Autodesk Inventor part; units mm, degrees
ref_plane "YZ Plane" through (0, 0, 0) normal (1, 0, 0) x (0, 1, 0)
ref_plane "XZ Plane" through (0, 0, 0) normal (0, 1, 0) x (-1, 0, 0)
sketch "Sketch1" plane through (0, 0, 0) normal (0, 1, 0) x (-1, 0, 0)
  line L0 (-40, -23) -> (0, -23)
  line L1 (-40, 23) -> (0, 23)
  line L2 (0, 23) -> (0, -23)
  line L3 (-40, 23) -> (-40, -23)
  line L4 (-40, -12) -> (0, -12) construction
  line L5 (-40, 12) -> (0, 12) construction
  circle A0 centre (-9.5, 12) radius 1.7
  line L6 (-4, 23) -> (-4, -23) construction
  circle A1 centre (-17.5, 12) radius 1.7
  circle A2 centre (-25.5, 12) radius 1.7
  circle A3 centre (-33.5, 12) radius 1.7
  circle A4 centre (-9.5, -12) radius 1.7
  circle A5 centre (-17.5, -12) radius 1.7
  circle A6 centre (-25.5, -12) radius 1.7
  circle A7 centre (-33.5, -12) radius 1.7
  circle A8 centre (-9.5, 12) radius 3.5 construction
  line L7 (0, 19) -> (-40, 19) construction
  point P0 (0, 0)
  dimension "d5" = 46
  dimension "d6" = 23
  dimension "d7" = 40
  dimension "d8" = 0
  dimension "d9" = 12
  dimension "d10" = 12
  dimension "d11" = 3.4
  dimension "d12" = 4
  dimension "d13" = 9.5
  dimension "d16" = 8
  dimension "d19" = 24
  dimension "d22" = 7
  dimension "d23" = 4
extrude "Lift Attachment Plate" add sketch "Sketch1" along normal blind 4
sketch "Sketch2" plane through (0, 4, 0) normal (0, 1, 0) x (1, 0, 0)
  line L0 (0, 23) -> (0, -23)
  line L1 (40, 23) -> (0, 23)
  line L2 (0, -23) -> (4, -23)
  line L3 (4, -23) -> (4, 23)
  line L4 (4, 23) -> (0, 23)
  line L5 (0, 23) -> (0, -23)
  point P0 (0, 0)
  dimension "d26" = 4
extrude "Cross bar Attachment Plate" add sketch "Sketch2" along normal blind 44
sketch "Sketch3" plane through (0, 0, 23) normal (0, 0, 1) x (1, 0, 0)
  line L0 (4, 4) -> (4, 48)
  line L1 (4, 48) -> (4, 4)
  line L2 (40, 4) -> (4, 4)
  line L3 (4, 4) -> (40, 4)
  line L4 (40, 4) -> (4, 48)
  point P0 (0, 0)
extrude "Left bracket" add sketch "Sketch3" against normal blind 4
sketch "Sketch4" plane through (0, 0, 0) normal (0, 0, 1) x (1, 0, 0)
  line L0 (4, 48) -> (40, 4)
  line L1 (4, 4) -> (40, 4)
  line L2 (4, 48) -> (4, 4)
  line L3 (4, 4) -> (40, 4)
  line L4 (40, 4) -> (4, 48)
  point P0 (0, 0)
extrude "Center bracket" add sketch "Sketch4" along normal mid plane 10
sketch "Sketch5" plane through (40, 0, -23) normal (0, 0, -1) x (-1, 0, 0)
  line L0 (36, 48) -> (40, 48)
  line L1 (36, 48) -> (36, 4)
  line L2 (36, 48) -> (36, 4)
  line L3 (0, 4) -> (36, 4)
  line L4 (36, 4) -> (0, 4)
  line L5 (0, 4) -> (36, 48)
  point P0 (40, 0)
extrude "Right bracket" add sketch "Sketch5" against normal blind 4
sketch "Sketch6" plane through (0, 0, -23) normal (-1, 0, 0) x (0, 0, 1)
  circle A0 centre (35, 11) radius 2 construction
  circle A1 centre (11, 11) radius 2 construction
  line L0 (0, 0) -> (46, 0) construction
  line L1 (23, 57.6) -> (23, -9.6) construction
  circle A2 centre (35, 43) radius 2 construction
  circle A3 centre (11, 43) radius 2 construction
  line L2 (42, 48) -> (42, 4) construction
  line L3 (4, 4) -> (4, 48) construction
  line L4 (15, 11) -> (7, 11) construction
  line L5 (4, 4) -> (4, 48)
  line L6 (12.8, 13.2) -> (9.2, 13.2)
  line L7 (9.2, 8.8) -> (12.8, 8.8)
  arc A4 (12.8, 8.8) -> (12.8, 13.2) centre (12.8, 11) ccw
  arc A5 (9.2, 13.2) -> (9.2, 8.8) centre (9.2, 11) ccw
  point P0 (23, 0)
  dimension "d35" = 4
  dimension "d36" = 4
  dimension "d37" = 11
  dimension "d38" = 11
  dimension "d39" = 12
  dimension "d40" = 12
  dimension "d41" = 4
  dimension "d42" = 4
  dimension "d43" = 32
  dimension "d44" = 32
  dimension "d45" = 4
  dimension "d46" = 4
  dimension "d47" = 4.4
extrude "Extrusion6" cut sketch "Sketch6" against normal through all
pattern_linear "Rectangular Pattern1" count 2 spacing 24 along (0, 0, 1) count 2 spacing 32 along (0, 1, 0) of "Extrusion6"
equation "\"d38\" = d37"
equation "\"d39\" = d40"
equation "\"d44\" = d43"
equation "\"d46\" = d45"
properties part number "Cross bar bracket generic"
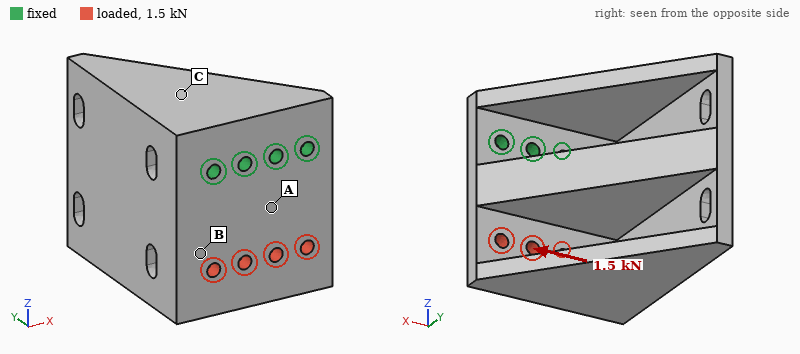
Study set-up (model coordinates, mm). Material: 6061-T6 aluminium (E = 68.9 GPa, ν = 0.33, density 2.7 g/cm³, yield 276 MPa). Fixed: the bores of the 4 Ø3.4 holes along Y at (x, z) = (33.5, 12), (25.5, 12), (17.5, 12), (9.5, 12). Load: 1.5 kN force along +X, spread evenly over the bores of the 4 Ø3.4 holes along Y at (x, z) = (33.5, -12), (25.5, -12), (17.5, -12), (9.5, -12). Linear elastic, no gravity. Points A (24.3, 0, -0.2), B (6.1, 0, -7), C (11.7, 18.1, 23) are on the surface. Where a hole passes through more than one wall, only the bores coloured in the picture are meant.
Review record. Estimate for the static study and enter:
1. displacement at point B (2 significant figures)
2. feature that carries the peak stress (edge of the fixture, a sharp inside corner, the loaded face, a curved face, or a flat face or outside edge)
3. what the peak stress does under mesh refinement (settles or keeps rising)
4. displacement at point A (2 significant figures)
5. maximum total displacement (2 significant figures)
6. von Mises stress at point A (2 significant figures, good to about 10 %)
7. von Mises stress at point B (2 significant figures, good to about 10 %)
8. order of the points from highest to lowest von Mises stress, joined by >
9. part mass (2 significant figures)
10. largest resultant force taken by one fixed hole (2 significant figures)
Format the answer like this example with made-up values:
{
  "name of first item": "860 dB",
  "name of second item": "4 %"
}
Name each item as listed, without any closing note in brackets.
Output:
{
  "displacement at point B": "13 µm",
  "feature that carries the peak stress": "edge of the fixture",
  "what the peak stress does under mesh refinement": "keeps rising",
  "displacement at point A": "7.1 µm",
  "maximum total displacement": "23 µm",
  "von Mises stress at point A": "21 MPa",
  "von Mises stress at point B": "13 MPa",
  "order of the points from highest to lowest von Mises stress, joined by >": "A > B > C",
  "part mass": "78 g",
  "largest resultant force taken by one fixed hole": "1.4 kN"
}
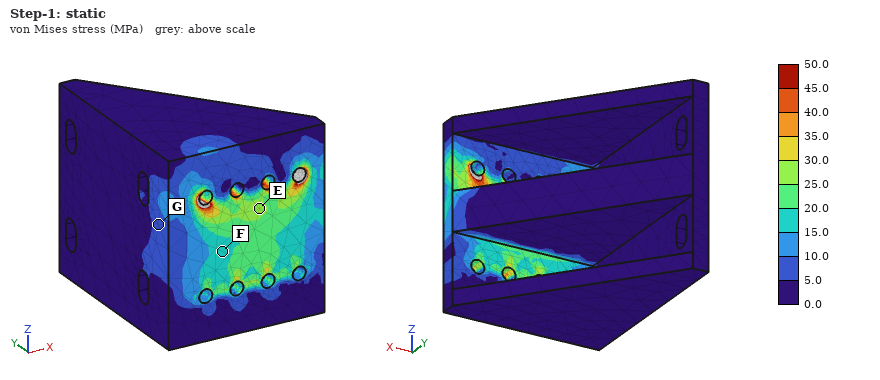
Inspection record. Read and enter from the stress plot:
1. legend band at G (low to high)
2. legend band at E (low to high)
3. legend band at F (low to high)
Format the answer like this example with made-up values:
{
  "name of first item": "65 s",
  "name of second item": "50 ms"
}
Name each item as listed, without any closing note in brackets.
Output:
{
  "legend band at G": "5.0 to 10.0 MPa",
  "legend band at E": "25.0 to 30.0 MPa",
  "legend band at F": "15.0 to 20.0 MPa"
}
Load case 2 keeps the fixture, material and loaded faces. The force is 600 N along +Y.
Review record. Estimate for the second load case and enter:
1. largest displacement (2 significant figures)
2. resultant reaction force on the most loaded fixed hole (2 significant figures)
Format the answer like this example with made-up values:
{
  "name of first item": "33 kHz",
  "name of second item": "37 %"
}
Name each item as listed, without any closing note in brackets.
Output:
{
  "largest displacement": "0.14 mm",
  "resultant reaction force on the most loaded fixed hole": "170 N"
}
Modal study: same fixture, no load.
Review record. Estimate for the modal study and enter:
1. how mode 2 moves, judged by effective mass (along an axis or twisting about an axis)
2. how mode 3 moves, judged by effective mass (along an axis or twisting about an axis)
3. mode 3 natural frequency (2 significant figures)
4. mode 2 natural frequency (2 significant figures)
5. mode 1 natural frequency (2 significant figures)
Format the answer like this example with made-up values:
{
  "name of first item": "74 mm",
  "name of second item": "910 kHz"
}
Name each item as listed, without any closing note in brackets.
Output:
{
  "how mode 2 moves, judged by effective mass": "along X",
  "how mode 3 moves, judged by effective mass": "along Y",
  "mode 3 natural frequency": "6800 Hz",
  "mode 2 natural frequency": "3900 Hz",
  "mode 1 natural frequency": "1600 Hz"
}
